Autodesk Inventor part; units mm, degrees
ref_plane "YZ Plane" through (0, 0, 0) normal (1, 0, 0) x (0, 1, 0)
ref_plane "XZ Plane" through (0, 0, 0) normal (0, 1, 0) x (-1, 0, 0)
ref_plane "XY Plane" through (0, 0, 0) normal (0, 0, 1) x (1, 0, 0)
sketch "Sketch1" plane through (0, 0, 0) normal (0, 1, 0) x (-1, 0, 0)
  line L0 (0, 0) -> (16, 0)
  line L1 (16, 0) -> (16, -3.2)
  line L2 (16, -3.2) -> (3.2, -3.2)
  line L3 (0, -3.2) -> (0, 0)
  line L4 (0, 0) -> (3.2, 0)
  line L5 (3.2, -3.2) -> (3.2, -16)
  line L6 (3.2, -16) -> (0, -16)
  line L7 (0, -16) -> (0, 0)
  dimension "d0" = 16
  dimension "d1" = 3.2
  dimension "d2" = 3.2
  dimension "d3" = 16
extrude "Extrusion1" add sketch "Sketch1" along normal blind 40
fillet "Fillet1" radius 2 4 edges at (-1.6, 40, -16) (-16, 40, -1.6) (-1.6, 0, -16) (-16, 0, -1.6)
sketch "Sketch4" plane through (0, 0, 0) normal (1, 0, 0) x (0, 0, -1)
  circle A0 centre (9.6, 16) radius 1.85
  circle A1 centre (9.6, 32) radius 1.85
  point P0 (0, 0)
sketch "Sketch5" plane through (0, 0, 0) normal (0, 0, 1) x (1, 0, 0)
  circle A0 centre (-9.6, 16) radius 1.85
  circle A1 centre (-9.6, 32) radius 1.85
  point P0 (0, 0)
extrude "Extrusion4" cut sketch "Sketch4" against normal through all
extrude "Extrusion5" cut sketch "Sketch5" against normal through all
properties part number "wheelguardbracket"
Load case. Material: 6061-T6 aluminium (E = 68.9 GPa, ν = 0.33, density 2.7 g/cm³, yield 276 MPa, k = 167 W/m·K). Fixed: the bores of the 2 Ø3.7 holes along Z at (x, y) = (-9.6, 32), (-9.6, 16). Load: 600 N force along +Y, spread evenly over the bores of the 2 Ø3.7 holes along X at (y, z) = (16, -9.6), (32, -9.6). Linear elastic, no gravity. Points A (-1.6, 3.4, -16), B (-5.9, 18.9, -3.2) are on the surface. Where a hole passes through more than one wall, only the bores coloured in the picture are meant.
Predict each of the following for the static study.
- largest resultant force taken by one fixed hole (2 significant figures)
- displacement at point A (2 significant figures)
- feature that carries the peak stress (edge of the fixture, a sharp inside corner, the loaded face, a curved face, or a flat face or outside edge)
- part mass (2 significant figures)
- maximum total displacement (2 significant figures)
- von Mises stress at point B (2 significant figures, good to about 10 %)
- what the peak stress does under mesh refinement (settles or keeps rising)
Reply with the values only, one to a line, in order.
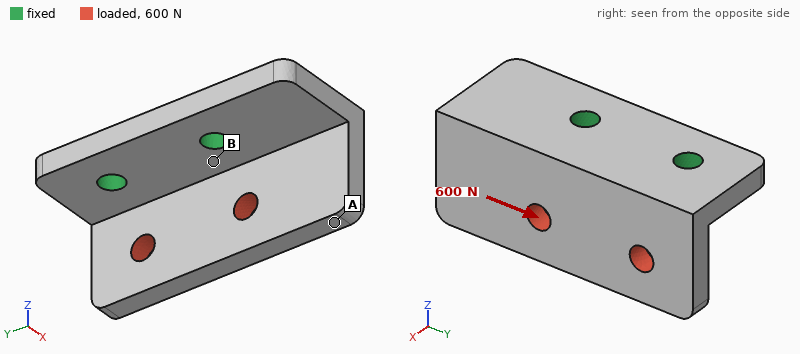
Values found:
450 N
30 µm
edge of the fixture
9.6 g
32 µm
33 MPa
keeps rising
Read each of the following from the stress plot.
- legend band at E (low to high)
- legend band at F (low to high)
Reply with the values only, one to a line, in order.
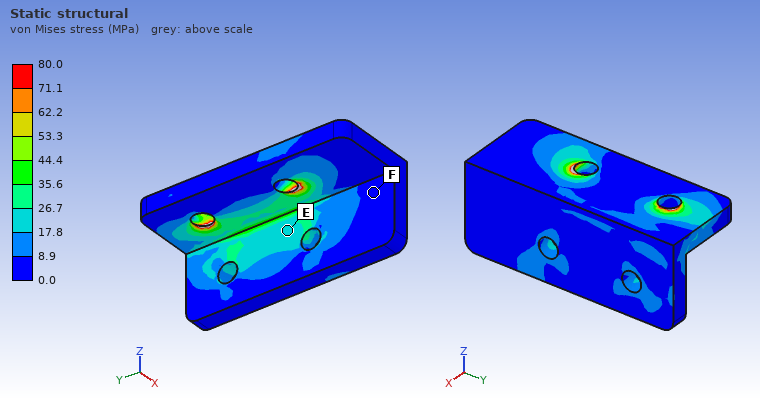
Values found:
17.8 to 26.7 MPa
0.0 to 8.9 MPa
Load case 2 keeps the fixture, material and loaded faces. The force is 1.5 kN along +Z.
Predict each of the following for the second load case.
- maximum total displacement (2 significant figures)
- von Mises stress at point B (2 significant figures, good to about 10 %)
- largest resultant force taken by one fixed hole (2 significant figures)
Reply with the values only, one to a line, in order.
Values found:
0.12 mm
100 MPa
750 N
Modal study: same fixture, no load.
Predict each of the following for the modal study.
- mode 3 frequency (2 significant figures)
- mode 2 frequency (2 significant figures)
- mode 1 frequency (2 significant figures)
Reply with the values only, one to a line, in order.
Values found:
13 kHz
9000 Hz
6500 Hz
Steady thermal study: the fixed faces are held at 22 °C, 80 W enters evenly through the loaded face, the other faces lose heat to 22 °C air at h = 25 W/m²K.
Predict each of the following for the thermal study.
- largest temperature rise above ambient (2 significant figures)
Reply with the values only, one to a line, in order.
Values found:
80 K
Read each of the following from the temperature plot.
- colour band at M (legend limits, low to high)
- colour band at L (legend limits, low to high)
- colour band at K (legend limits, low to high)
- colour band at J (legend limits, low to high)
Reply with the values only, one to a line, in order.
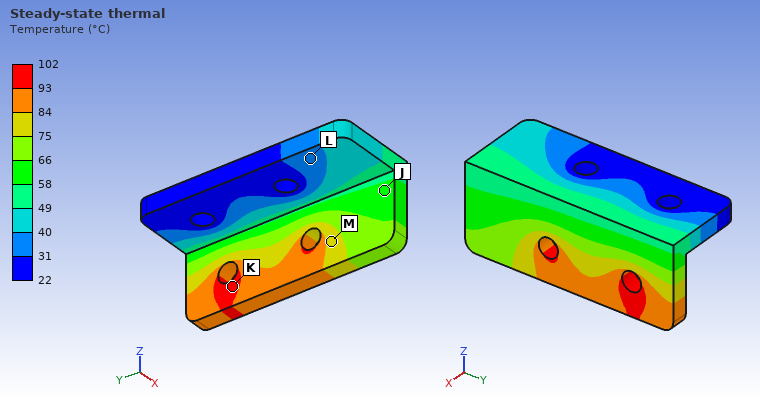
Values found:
75 to 84 °C
31 to 40 °C
93 to 102 °C
58 to 66 °C
